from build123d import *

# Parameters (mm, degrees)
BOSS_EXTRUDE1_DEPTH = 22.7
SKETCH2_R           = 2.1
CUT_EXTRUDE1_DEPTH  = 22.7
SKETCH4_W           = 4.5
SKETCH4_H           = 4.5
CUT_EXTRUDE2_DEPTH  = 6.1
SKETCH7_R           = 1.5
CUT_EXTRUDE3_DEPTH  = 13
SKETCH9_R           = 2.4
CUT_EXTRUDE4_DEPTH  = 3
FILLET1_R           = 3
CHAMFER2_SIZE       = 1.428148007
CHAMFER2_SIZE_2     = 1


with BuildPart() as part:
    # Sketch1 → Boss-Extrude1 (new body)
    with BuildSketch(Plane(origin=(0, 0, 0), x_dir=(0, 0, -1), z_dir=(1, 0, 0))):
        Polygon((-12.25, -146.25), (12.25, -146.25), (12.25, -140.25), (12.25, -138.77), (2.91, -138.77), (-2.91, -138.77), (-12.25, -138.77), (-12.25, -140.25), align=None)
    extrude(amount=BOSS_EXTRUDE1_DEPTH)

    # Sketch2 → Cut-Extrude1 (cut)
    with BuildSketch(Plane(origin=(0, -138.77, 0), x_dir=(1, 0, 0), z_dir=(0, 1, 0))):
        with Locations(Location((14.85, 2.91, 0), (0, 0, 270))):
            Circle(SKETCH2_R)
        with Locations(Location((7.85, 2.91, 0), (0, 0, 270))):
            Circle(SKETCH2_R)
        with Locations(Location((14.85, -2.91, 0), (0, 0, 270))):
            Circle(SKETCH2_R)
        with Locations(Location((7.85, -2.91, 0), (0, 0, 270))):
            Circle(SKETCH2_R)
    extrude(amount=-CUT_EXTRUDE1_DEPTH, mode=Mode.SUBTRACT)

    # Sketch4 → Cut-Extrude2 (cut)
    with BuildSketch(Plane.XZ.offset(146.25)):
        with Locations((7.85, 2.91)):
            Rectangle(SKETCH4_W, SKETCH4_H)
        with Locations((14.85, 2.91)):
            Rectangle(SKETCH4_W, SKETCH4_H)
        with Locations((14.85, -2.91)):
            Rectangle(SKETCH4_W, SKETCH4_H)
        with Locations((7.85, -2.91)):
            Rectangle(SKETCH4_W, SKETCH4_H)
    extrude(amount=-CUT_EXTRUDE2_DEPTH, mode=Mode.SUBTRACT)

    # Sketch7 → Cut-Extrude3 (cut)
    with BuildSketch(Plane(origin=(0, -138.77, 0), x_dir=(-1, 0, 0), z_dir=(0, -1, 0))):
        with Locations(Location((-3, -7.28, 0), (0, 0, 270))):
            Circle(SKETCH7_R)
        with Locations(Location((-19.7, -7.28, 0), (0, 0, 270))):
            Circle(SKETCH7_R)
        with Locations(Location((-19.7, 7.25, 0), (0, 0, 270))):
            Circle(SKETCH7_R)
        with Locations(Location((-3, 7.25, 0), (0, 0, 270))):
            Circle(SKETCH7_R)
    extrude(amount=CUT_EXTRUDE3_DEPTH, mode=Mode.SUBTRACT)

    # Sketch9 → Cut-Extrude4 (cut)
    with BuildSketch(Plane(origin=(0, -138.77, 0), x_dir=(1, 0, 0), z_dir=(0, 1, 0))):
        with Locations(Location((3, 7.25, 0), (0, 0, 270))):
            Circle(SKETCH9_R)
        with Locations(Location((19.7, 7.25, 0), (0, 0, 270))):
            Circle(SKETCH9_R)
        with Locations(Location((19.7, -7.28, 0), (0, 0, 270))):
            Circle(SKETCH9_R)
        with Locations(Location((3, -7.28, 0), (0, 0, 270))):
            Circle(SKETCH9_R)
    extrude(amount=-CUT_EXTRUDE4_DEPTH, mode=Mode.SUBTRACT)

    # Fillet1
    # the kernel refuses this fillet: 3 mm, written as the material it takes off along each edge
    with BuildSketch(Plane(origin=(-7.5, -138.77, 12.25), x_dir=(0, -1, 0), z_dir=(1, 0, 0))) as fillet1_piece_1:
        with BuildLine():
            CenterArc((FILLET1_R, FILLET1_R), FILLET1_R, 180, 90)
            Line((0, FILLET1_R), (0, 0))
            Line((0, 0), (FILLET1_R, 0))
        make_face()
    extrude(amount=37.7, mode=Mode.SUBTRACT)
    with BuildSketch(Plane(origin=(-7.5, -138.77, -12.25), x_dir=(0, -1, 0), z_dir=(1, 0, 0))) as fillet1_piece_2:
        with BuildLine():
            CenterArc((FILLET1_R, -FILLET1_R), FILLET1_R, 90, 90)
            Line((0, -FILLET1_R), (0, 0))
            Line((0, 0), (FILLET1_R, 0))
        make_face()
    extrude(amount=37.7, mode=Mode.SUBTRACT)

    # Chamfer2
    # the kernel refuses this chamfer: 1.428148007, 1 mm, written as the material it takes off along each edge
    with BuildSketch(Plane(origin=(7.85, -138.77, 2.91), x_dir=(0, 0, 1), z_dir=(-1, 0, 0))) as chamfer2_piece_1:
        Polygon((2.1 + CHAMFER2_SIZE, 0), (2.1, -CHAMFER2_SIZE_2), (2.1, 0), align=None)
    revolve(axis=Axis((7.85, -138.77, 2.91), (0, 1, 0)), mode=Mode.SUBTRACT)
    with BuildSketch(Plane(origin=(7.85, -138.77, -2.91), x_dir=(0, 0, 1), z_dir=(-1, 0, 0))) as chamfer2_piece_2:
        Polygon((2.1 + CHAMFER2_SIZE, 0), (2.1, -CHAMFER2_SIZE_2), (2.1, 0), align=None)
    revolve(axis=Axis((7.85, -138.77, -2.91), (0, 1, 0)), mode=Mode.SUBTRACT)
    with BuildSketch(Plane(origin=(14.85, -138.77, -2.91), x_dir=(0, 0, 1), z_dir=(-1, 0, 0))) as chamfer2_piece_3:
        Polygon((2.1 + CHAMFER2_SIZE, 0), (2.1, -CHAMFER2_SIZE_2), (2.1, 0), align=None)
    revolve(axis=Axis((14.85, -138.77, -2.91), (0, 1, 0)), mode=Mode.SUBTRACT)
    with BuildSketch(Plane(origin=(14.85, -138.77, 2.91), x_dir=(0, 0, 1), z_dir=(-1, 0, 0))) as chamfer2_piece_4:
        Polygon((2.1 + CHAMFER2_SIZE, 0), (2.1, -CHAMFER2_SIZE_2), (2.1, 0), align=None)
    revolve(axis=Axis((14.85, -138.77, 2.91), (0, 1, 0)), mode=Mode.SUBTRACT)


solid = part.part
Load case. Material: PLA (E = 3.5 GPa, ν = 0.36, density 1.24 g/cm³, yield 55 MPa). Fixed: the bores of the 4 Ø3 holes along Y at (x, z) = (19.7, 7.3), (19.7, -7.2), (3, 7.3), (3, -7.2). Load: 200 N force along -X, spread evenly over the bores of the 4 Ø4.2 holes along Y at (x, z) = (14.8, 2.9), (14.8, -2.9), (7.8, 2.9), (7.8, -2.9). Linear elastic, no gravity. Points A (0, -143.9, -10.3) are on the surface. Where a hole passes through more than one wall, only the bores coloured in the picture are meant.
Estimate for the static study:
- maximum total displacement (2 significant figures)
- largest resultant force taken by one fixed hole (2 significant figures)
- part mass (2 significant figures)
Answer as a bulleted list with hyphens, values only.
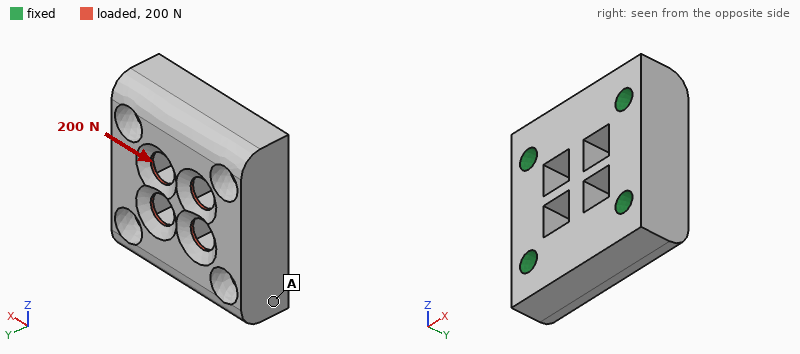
- 15 µm
- 55 N
- 3.9 g
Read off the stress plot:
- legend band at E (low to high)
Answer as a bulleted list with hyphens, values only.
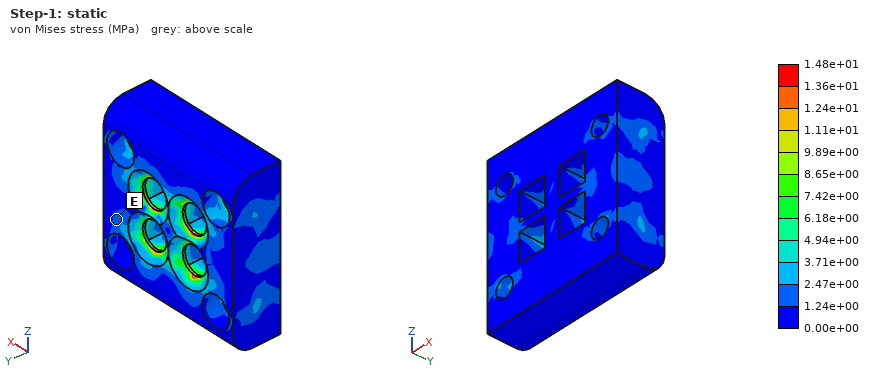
- 1.24e+00 to 2.47e+00 MPa
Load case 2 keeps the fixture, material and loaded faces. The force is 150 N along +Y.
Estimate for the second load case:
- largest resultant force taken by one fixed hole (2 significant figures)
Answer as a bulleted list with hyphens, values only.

- 41 N
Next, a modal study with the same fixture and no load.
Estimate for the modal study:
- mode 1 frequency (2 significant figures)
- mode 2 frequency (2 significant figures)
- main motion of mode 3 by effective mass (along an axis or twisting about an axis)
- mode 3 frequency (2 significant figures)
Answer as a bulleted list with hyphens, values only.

- 19 kHz
- 20 kHz
- along Z
- 22 kHz
